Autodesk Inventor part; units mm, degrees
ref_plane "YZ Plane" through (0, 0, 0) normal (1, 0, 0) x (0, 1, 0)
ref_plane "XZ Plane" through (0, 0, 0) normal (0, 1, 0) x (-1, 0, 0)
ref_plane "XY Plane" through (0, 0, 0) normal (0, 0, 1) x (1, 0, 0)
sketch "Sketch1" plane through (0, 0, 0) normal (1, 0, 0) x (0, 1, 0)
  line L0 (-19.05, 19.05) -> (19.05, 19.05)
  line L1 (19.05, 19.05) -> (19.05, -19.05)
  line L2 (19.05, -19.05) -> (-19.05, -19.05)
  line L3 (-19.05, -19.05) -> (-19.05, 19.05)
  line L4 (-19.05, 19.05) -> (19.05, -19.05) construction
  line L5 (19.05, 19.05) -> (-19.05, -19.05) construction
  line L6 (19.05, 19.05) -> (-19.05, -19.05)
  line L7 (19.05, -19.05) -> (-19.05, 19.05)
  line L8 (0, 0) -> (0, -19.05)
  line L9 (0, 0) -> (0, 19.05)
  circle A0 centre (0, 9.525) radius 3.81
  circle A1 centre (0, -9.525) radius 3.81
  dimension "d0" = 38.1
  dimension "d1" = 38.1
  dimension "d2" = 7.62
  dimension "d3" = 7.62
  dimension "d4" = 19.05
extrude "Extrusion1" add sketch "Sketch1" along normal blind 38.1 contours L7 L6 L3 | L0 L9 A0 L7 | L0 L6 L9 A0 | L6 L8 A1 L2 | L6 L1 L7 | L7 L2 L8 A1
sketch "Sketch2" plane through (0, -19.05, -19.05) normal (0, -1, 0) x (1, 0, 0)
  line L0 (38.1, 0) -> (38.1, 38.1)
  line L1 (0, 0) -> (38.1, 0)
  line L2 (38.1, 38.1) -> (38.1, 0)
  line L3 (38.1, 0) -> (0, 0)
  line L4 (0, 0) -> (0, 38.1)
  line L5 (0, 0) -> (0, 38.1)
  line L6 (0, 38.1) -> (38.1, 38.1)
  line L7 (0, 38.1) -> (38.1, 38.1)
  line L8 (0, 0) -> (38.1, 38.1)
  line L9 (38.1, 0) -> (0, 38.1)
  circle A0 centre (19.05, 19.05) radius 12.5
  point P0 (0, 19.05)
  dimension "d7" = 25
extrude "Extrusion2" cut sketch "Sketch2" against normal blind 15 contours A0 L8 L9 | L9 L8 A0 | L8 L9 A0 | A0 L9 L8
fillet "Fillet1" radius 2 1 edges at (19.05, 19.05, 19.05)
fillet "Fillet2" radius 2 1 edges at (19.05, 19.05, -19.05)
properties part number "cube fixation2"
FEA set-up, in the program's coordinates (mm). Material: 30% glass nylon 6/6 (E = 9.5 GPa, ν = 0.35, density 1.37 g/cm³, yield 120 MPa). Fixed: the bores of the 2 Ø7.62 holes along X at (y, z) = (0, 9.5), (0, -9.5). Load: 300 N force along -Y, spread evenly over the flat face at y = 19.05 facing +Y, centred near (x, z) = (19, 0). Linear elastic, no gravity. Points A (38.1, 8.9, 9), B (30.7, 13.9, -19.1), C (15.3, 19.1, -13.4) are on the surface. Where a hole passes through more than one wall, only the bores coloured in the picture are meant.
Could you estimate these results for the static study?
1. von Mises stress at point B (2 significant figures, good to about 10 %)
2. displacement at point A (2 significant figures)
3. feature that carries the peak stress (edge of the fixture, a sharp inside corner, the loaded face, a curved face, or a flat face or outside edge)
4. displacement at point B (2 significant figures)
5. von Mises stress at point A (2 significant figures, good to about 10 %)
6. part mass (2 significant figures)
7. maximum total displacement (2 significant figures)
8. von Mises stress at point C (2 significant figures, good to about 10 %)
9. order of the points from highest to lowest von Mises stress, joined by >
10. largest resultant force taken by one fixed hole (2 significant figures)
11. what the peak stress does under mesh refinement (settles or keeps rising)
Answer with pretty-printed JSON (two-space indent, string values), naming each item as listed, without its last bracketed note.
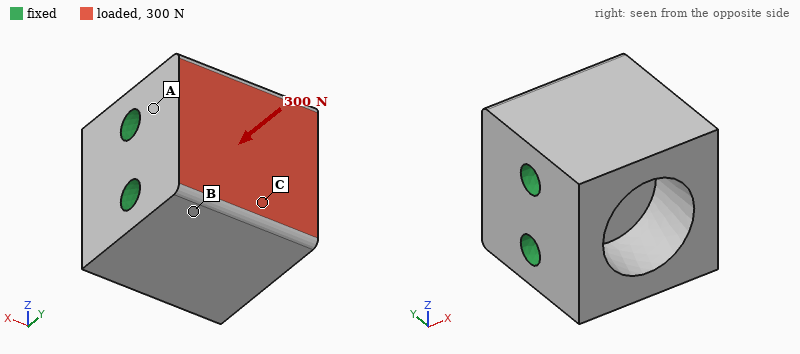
{
  "von Mises stress at point B": "0.073 MPa",
  "displacement at point A": "0.23 µm",
  "feature that carries the peak stress": "edge of the fixture",
  "displacement at point B": "0.30 µm",
  "von Mises stress at point A": "0.27 MPa",
  "part mass": "61 g",
  "maximum total displacement": "0.48 µm",
  "von Mises stress at point C": "0.18 MPa",
  "order of the points from highest to lowest von Mises stress, joined by >": "A > C > B",
  "largest resultant force taken by one fixed hole": "150 N",
  "what the peak stress does under mesh refinement": "keeps rising"
}
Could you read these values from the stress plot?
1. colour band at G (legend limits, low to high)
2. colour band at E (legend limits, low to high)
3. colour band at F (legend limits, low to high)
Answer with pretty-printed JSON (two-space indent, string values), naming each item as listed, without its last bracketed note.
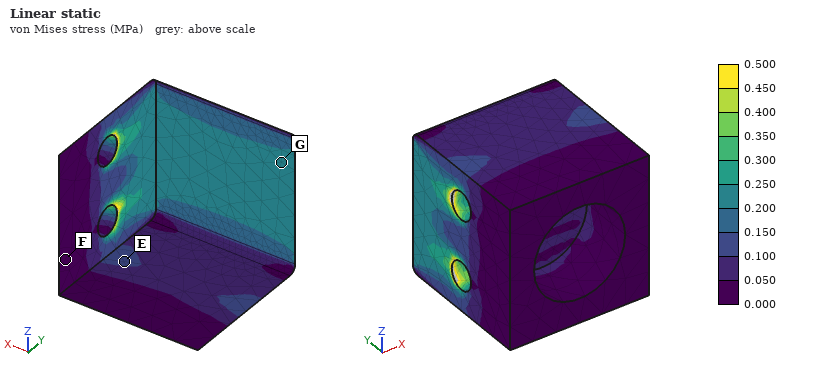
{
  "colour band at G": "0.200 to 0.250 MPa",
  "colour band at E": "0.100 to 0.150 MPa",
  "colour band at F": "0.000 to 0.050 MPa"
}
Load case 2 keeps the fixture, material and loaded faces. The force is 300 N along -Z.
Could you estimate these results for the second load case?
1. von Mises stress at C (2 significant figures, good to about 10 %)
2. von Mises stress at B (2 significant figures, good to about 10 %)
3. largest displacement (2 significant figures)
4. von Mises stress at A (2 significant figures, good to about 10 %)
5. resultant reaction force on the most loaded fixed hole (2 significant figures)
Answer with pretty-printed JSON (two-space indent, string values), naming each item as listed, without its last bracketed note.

{
  "von Mises stress at C": "0.44 MPa",
  "von Mises stress at B": "0.22 MPa",
  "largest displacement": "2.0 µm",
  "von Mises stress at A": "0.42 MPa",
  "resultant reaction force on the most loaded fixed hole": "250 N"
}
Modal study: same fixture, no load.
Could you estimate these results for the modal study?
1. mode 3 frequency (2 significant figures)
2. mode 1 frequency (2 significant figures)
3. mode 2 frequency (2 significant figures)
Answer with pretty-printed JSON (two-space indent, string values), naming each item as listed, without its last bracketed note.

{
  "mode 3 frequency": "17 kHz",
  "mode 1 frequency": "15 kHz",
  "mode 2 frequency": "17 kHz"
}
